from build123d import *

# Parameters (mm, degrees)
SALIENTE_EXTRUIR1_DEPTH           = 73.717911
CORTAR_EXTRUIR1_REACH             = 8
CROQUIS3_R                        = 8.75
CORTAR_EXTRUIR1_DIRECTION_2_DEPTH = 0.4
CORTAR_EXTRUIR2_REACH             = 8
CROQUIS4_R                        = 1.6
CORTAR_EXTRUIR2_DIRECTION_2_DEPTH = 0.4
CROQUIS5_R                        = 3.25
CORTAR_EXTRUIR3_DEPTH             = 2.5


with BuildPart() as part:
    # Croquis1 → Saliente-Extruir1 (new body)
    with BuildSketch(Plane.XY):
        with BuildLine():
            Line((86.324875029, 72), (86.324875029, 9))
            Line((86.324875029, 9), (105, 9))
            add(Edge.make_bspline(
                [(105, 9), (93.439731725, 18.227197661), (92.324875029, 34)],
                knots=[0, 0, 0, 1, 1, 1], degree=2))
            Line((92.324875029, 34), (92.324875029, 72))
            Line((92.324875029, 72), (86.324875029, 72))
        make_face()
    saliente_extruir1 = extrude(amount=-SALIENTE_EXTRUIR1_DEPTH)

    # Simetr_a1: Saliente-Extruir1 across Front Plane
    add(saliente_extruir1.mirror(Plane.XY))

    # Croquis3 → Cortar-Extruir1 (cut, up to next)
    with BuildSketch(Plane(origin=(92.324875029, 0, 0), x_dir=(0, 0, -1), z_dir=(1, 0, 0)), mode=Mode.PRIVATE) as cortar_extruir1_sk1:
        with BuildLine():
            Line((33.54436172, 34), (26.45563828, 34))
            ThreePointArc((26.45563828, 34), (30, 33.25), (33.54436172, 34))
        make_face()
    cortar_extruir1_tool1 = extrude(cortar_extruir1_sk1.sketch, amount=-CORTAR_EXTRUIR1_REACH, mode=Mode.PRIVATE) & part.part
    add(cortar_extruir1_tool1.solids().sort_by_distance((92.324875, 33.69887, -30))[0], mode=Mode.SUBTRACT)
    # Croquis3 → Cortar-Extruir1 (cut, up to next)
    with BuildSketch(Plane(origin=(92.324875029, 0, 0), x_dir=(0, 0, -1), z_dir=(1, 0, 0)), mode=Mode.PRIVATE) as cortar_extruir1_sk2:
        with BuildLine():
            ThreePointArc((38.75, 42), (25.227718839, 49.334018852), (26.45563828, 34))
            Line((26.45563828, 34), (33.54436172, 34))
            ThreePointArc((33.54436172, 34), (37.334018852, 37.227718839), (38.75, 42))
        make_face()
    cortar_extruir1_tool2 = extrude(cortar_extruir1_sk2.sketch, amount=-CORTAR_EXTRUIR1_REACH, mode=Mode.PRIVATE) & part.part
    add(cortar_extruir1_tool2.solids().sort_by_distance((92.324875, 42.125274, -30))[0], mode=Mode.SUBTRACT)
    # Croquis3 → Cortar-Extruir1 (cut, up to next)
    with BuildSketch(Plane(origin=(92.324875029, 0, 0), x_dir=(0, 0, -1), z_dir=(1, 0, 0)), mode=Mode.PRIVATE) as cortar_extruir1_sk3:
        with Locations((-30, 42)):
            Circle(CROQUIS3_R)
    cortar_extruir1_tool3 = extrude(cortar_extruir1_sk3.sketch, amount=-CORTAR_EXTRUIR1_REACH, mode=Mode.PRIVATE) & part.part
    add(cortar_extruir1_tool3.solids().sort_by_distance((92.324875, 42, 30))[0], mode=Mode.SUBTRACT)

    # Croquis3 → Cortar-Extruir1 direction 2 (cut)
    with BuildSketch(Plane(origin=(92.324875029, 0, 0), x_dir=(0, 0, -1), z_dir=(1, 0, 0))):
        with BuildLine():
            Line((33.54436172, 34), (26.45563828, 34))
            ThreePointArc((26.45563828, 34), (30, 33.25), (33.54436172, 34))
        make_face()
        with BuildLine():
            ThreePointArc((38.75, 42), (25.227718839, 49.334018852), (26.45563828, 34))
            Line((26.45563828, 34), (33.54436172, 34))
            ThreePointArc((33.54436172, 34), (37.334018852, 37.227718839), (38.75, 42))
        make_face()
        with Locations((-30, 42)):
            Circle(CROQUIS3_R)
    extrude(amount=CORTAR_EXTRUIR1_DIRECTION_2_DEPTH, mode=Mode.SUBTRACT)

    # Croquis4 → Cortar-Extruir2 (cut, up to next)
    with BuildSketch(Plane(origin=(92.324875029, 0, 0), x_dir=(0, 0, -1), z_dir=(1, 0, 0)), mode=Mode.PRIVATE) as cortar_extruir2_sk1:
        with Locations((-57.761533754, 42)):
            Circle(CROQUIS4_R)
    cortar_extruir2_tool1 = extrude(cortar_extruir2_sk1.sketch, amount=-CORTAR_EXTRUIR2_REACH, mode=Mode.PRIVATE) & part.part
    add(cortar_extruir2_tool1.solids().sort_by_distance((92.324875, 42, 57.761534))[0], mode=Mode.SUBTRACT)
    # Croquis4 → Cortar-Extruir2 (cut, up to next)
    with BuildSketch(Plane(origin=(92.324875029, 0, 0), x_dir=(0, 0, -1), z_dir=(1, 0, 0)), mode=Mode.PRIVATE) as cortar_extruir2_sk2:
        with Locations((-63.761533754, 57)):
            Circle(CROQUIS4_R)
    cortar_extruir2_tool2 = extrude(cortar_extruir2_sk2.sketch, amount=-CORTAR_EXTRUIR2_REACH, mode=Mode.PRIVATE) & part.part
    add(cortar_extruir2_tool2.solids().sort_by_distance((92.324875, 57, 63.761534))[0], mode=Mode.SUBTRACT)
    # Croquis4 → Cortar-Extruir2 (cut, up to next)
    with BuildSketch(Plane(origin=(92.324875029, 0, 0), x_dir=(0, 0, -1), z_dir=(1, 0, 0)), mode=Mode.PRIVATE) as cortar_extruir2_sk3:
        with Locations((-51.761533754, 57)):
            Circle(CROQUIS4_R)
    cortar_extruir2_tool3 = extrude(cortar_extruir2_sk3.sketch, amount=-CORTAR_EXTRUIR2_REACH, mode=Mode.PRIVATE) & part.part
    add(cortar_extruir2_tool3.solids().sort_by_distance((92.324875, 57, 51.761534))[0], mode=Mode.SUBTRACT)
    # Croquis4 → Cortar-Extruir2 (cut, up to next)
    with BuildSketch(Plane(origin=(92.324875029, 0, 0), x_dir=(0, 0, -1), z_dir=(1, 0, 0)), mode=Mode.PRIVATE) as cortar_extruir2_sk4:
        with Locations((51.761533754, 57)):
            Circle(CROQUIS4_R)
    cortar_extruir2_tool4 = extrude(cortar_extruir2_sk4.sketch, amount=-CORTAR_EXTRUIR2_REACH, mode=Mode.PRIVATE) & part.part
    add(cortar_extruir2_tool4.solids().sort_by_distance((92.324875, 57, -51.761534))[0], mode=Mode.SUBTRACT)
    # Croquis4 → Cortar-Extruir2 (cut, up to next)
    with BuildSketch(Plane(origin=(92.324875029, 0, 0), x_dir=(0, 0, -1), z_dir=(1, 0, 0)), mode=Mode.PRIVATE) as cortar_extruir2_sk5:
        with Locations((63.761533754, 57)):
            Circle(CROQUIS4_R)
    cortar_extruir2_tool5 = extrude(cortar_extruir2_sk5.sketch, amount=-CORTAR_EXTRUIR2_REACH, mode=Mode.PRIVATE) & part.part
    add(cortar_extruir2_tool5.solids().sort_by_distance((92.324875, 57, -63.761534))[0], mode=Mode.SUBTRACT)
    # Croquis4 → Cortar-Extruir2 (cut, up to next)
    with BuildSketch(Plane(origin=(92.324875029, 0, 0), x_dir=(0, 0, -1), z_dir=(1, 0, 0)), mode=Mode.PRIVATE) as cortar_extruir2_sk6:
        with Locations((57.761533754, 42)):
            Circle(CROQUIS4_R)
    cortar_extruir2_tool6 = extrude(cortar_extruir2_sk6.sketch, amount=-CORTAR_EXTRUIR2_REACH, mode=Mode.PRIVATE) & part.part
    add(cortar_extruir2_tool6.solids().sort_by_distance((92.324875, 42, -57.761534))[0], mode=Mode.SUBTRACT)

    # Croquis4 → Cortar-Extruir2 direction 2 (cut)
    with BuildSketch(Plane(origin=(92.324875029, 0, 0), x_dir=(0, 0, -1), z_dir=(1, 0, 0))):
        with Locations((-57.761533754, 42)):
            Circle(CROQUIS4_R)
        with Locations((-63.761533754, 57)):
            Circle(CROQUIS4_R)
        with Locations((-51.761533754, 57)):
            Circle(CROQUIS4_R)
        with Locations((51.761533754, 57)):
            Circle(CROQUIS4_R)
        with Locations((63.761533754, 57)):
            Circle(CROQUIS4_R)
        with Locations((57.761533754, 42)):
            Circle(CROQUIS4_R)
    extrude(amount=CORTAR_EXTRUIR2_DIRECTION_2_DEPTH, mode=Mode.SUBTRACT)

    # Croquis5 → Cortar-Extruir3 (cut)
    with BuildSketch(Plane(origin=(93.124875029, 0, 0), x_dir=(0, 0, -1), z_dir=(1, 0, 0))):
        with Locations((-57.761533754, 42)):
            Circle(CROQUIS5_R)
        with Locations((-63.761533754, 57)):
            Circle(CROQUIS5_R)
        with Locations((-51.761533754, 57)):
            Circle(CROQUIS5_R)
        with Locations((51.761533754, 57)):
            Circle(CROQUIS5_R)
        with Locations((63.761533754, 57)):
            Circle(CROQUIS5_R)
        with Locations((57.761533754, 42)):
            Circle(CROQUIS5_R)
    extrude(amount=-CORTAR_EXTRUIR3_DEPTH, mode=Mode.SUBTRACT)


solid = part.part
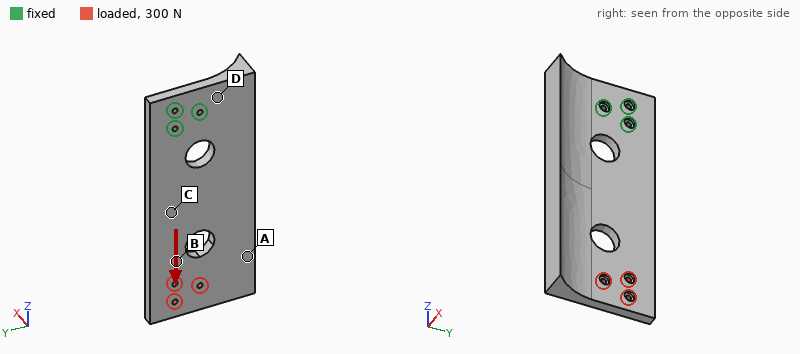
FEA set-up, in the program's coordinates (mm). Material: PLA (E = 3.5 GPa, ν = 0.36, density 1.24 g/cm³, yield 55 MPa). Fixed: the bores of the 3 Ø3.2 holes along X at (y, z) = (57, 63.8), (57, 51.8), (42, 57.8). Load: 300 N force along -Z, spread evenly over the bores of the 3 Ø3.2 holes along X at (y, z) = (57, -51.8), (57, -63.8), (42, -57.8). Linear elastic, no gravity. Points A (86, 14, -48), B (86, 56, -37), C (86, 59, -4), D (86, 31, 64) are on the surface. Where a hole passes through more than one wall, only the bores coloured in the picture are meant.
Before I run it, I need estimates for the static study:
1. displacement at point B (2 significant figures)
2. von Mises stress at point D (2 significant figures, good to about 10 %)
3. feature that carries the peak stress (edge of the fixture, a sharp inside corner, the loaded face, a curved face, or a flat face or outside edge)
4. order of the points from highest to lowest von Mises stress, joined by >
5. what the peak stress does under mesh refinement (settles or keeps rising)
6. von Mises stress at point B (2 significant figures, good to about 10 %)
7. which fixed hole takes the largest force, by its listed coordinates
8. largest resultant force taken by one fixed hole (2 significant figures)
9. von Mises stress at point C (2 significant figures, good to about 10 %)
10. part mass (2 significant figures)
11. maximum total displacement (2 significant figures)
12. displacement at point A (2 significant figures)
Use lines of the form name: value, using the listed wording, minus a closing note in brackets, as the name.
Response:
displacement at point B: 0.15 mm
von Mises stress at point D: 0.78 MPa
feature that carries the peak stress: edge of the fixture
order of the points from highest to lowest von Mises stress, joined by >: B > C > D > A
what the peak stress does under mesh refinement: keeps rising
von Mises stress at point B: 2.4 MPa
which fixed hole takes the largest force, by its listed coordinates: (57, 51.8)
largest resultant force taken by one fixed hole: 140 N
von Mises stress at point C: 1.7 MPa
part mass: 83 g
maximum total displacement: 0.29 mm
displacement at point A: 0.18 mm
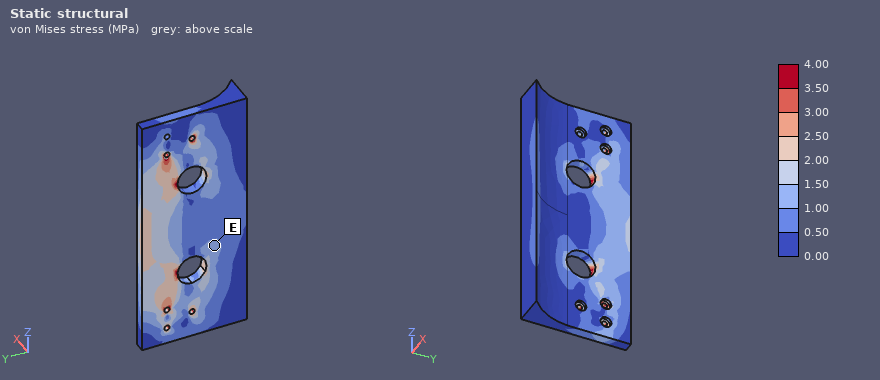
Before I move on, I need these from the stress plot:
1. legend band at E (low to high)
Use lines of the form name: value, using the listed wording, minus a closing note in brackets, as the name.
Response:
legend band at E: 1.00 to 1.50 MPa
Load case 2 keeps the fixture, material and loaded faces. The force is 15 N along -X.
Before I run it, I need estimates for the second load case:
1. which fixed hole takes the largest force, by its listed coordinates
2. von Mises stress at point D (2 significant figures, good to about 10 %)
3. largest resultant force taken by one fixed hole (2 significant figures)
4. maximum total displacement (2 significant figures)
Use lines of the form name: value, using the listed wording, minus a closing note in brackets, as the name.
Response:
which fixed hole takes the largest force, by its listed coordinates: (57, 51.8)
von Mises stress at point D: 2.6 MPa
largest resultant force taken by one fixed hole: 77 N
maximum total displacement: 1.5 mm
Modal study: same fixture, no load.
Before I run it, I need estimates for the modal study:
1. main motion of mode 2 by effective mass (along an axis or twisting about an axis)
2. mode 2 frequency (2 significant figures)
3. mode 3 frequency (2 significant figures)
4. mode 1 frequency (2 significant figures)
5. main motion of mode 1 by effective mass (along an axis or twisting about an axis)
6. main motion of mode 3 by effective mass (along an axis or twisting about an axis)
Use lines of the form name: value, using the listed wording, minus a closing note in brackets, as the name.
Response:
main motion of mode 2 by effective mass: twisting about Z
mode 2 frequency: 340 Hz
mode 3 frequency: 430 Hz
mode 1 frequency: 100 Hz
main motion of mode 1 by effective mass: along X
main motion of mode 3 by effective mass: along Y
